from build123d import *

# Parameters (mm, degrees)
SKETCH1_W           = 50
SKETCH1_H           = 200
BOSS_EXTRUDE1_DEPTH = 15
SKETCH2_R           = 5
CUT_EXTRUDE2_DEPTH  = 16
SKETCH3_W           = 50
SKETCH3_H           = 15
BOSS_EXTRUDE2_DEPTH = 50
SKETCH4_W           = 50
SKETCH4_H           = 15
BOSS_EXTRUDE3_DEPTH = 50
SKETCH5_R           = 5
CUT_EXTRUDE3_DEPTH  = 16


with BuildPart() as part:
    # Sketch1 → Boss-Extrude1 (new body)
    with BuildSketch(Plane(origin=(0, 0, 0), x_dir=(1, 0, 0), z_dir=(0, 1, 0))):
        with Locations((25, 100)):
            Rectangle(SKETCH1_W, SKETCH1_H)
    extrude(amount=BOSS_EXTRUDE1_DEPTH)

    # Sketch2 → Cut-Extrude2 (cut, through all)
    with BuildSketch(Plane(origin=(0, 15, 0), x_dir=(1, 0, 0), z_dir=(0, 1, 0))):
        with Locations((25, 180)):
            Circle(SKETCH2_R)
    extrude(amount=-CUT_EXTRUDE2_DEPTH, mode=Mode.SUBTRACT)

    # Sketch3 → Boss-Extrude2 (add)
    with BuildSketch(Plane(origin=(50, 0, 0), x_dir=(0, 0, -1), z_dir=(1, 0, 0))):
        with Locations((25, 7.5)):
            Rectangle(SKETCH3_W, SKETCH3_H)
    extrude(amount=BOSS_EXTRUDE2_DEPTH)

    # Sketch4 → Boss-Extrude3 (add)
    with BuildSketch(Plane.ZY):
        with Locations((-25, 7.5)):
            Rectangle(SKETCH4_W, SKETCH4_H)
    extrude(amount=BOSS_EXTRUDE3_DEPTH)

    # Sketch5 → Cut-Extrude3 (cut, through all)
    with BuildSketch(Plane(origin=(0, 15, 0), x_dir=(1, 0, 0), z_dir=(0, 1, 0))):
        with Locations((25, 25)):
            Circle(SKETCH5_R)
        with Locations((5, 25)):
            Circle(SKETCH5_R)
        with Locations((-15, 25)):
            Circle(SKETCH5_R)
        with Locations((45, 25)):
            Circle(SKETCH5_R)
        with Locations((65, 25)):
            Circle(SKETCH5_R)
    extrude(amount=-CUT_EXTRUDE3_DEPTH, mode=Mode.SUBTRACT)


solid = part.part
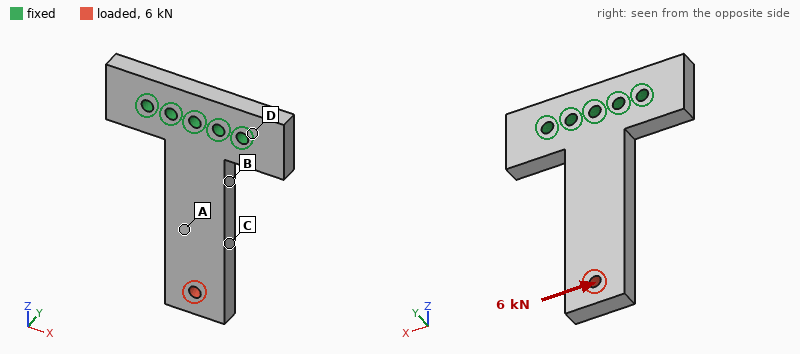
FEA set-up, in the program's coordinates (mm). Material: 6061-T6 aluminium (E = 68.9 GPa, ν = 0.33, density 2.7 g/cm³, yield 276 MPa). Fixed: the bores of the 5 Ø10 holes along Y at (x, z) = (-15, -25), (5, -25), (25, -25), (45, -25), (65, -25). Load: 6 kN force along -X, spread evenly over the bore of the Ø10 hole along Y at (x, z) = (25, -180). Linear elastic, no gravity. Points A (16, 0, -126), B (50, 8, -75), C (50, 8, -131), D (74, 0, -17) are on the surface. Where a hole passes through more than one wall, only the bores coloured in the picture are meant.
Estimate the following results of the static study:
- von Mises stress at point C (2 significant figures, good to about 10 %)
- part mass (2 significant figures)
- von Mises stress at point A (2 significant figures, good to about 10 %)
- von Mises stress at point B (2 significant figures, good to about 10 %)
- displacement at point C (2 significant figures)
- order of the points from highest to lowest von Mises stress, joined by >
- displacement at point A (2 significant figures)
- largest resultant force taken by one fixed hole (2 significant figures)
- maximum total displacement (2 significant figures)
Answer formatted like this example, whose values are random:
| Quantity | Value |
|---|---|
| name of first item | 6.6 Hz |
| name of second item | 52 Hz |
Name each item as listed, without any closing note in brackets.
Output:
| Quantity | Value |
|---|---|
| von Mises stress at point C | 47 MPa |
| part mass | 590 g |
| von Mises stress at point A | 26 MPa |
| von Mises stress at point B | 100 MPa |
| displacement at point C | 0.32 mm |
| order of the points from highest to lowest von Mises stress, joined by > | B > C > A > D |
| displacement at point A | 0.27 mm |
| largest resultant force taken by one fixed hole | 11 kN |
| maximum total displacement | 0.71 mm |
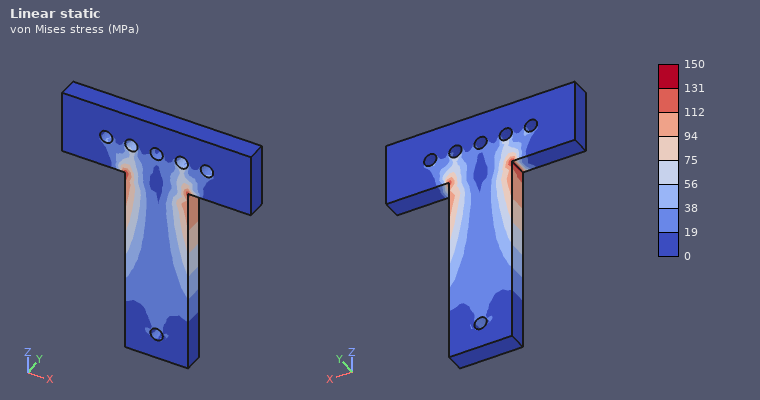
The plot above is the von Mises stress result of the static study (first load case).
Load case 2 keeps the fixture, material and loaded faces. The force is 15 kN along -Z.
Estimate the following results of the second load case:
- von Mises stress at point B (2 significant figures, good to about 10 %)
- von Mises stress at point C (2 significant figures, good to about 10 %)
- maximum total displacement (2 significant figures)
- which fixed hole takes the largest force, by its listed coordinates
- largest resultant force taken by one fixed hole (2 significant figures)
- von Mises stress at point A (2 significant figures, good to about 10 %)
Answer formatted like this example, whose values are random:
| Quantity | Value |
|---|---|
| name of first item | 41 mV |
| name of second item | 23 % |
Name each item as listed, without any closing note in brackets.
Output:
| Quantity | Value |
|---|---|
| von Mises stress at point B | 20 MPa |
| von Mises stress at point C | 20 MPa |
| maximum total displacement | 51 µm |
| which fixed hole takes the largest force, by its listed coordinates | (25, -25) |
| largest resultant force taken by one fixed hole | 4.9 kN |
| von Mises stress at point A | 20 MPa |
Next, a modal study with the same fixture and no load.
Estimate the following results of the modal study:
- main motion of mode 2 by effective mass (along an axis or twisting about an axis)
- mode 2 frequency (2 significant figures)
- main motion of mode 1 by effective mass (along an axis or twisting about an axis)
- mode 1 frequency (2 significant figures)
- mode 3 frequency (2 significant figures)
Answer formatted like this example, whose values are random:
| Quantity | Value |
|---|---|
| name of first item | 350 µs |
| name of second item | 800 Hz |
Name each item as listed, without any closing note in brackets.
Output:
| Quantity | Value |
|---|---|
| main motion of mode 2 by effective mass | along X |
| mode 2 frequency | 1500 Hz |
| main motion of mode 1 by effective mass | along Y |
| mode 1 frequency | 450 Hz |
| mode 3 frequency | 2600 Hz |
